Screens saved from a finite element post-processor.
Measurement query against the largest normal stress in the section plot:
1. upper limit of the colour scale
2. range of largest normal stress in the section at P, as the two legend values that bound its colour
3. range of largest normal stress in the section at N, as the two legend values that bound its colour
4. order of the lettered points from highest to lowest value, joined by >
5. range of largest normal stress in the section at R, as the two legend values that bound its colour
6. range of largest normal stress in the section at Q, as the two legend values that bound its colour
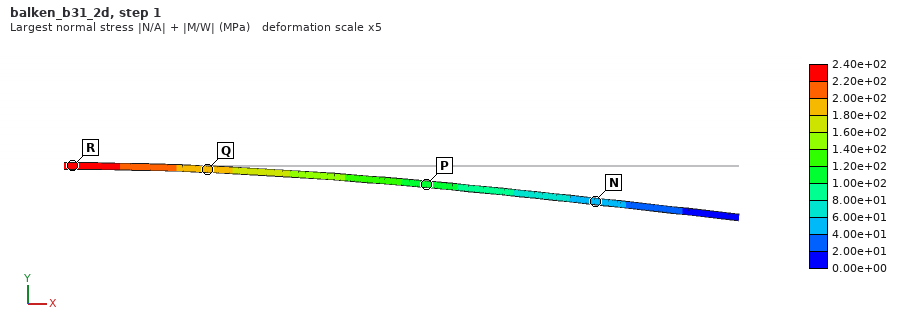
2.40e+02 MPa
1.00e+02 to 1.20e+02 MPa
4.00e+01 to 6.00e+01 MPa
R > Q > P > N
2.20e+02 to 2.40e+02 MPa
1.80e+02 to 2.00e+02 MPa
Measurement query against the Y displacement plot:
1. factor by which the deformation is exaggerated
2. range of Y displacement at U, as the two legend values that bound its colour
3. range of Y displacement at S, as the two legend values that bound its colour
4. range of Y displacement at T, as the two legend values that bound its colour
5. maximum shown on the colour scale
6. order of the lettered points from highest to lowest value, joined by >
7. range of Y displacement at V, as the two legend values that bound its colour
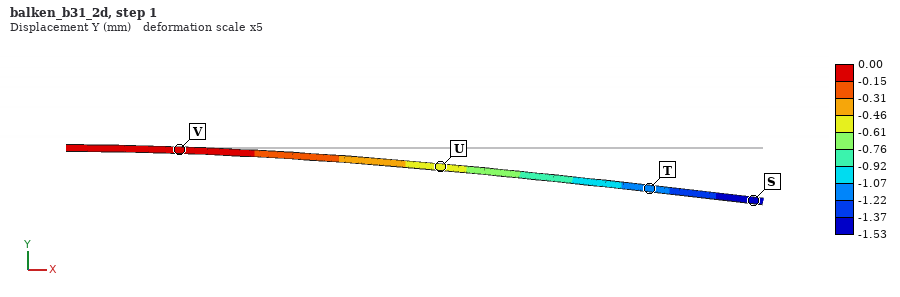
5
-0.61 to -0.46 mm
-1.53 to -1.37 mm
-1.22 to -1.07 mm
0.00 mm
V > U > T > S
-0.15 to 0.00 mm
